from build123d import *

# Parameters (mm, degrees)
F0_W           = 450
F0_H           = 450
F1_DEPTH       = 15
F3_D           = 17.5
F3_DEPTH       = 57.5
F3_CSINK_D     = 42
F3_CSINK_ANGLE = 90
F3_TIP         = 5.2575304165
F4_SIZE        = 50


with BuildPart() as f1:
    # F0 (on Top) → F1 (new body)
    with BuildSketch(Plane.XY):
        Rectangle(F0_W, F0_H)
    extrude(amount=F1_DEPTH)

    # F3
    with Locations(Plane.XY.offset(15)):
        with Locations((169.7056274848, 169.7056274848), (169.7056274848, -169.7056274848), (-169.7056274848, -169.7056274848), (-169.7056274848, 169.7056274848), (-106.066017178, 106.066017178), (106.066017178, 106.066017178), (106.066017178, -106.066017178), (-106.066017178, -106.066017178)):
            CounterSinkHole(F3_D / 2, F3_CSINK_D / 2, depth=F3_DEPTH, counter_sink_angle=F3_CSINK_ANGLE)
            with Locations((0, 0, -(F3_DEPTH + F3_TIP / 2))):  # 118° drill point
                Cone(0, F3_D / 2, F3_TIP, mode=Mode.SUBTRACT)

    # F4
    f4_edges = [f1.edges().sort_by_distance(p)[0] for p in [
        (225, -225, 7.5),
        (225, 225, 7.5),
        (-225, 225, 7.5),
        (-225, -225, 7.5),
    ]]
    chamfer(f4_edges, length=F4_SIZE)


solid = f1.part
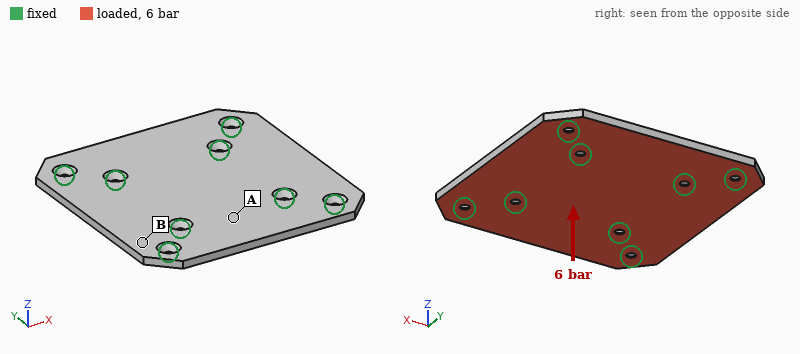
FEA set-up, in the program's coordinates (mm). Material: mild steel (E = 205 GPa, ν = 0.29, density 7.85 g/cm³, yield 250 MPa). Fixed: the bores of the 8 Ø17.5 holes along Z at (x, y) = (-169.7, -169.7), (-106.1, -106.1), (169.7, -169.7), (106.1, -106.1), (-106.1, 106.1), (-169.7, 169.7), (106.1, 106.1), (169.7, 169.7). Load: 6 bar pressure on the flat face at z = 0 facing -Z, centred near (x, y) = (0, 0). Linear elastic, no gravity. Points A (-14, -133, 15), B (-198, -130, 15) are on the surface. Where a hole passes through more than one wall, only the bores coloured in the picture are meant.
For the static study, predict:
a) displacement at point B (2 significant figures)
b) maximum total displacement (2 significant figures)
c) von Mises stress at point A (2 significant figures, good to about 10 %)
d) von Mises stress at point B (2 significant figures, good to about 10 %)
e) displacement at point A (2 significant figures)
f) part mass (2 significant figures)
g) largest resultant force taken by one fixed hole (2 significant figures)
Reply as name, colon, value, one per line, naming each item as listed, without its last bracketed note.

displacement at point B: 0.057 mm
maximum total displacement: 0.25 mm
von Mises stress at point A: 55 MPa
von Mises stress at point B: 22 MPa
displacement at point A: 0.13 mm
part mass: 23 kg
largest resultant force taken by one fixed hole: 23 kN
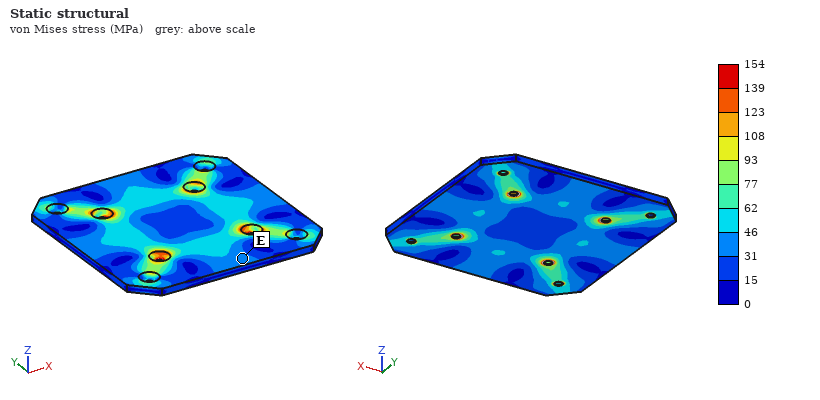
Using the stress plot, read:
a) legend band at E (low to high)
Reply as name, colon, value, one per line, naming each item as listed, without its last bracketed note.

legend band at E: 31 to 46 MPa
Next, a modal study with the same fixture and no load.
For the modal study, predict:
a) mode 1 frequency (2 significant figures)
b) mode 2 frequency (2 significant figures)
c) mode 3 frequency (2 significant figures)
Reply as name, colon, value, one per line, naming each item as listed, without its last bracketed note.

mode 1 frequency: 650 Hz
mode 2 frequency: 760 Hz
mode 3 frequency: 760 Hz
